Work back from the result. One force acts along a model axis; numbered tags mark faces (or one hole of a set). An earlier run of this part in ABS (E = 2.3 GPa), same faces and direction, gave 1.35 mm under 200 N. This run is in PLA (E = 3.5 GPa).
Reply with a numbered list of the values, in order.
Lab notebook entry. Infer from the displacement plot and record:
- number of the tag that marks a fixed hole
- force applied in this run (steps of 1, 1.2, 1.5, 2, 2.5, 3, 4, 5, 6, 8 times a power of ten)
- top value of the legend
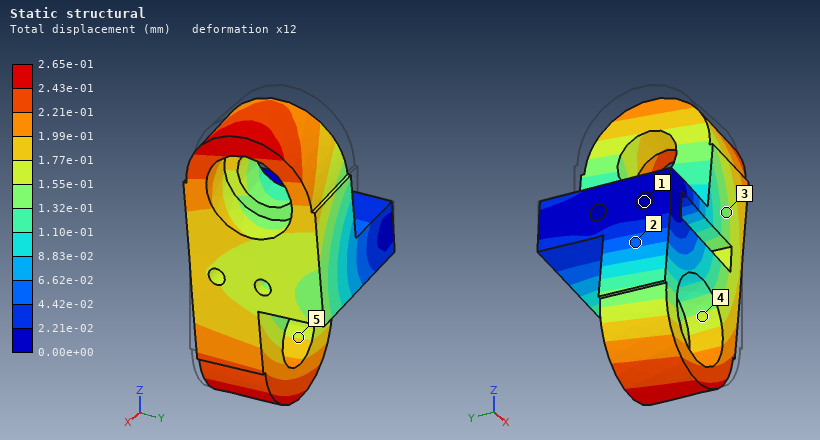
1. 1
2. 60 N
3. 2.65e-01 mm
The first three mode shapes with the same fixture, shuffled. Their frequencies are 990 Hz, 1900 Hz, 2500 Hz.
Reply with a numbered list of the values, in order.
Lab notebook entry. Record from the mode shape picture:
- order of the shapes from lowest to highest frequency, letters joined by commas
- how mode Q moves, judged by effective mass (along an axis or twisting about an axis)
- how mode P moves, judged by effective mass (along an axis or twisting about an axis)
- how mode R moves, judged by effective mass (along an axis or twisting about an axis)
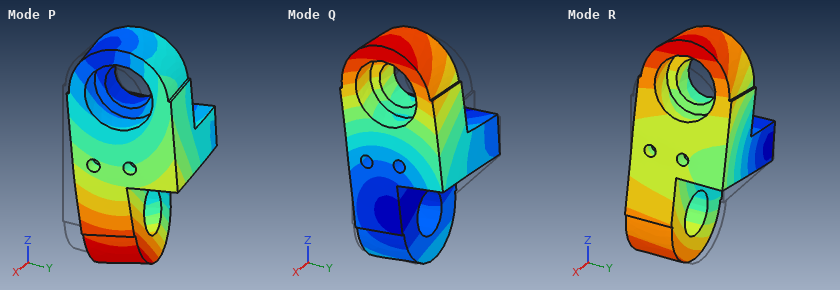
1. R, Q, P
2. along Y
3. along Y
4. along Z
